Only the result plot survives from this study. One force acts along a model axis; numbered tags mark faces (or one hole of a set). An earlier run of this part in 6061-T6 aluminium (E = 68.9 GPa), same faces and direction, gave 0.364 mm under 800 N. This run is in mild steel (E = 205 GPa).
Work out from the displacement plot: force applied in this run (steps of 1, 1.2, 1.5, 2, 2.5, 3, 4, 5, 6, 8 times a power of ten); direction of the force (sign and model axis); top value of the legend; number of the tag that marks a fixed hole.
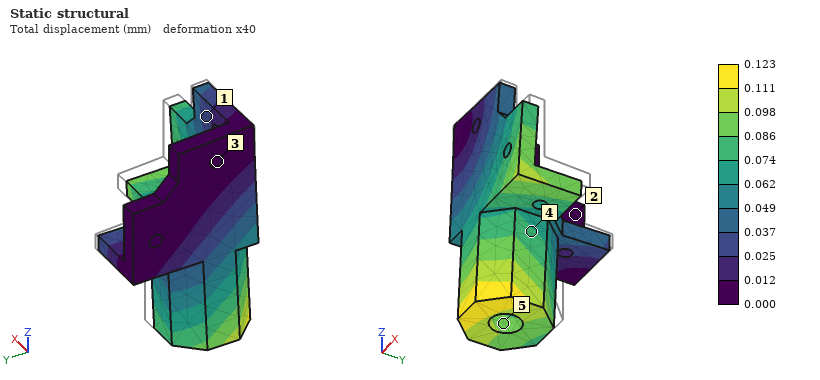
800 N
-X
0.123 mm
3
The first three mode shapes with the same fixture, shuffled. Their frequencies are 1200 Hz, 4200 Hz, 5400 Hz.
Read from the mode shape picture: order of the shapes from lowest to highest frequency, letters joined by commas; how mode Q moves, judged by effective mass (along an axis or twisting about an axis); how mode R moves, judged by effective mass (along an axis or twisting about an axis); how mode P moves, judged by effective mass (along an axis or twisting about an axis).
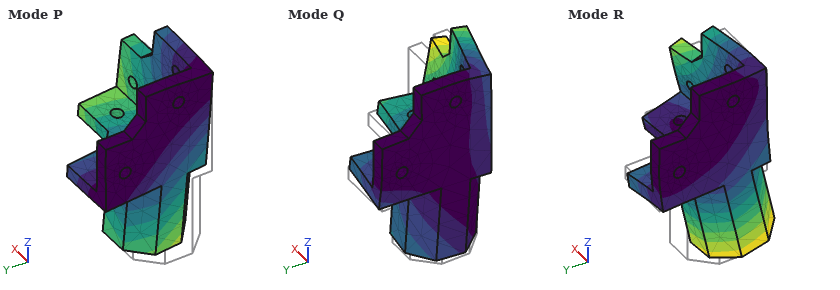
P, Q, R
along Y
along Y
along X
